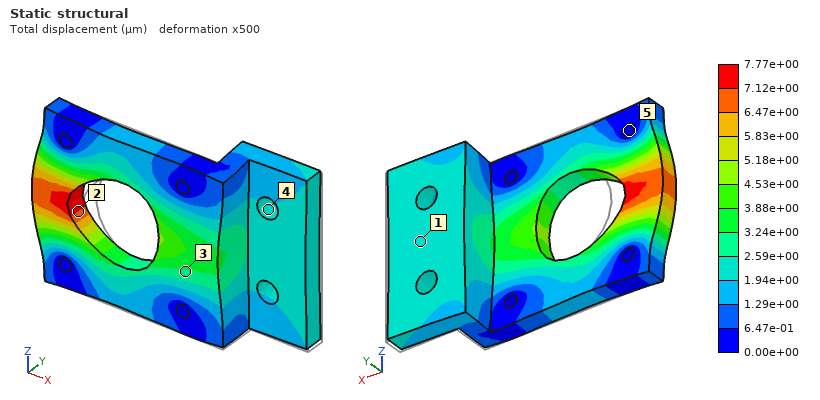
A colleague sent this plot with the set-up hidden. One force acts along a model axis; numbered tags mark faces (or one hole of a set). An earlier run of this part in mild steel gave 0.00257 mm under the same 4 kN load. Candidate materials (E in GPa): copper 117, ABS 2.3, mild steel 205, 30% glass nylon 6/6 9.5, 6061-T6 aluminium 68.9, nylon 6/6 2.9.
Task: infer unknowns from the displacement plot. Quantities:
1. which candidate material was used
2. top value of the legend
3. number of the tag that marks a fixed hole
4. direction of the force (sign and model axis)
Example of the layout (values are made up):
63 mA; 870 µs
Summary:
6061-T6 aluminium; 7.77e+00 µm; 5; -X
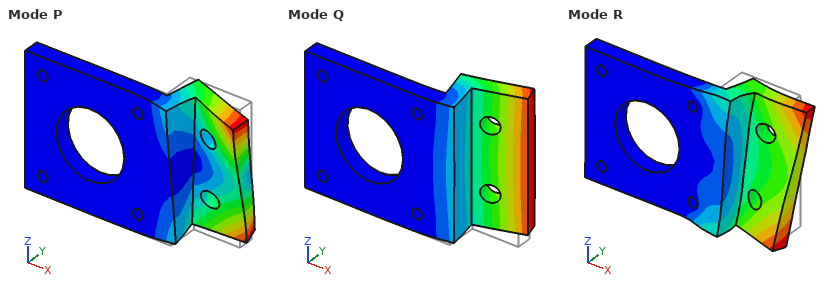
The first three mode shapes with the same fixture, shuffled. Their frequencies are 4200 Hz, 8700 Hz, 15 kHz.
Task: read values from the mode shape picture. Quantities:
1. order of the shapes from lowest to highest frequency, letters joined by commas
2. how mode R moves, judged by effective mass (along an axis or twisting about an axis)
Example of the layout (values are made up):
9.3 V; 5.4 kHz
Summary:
Q, P, R; along Z
